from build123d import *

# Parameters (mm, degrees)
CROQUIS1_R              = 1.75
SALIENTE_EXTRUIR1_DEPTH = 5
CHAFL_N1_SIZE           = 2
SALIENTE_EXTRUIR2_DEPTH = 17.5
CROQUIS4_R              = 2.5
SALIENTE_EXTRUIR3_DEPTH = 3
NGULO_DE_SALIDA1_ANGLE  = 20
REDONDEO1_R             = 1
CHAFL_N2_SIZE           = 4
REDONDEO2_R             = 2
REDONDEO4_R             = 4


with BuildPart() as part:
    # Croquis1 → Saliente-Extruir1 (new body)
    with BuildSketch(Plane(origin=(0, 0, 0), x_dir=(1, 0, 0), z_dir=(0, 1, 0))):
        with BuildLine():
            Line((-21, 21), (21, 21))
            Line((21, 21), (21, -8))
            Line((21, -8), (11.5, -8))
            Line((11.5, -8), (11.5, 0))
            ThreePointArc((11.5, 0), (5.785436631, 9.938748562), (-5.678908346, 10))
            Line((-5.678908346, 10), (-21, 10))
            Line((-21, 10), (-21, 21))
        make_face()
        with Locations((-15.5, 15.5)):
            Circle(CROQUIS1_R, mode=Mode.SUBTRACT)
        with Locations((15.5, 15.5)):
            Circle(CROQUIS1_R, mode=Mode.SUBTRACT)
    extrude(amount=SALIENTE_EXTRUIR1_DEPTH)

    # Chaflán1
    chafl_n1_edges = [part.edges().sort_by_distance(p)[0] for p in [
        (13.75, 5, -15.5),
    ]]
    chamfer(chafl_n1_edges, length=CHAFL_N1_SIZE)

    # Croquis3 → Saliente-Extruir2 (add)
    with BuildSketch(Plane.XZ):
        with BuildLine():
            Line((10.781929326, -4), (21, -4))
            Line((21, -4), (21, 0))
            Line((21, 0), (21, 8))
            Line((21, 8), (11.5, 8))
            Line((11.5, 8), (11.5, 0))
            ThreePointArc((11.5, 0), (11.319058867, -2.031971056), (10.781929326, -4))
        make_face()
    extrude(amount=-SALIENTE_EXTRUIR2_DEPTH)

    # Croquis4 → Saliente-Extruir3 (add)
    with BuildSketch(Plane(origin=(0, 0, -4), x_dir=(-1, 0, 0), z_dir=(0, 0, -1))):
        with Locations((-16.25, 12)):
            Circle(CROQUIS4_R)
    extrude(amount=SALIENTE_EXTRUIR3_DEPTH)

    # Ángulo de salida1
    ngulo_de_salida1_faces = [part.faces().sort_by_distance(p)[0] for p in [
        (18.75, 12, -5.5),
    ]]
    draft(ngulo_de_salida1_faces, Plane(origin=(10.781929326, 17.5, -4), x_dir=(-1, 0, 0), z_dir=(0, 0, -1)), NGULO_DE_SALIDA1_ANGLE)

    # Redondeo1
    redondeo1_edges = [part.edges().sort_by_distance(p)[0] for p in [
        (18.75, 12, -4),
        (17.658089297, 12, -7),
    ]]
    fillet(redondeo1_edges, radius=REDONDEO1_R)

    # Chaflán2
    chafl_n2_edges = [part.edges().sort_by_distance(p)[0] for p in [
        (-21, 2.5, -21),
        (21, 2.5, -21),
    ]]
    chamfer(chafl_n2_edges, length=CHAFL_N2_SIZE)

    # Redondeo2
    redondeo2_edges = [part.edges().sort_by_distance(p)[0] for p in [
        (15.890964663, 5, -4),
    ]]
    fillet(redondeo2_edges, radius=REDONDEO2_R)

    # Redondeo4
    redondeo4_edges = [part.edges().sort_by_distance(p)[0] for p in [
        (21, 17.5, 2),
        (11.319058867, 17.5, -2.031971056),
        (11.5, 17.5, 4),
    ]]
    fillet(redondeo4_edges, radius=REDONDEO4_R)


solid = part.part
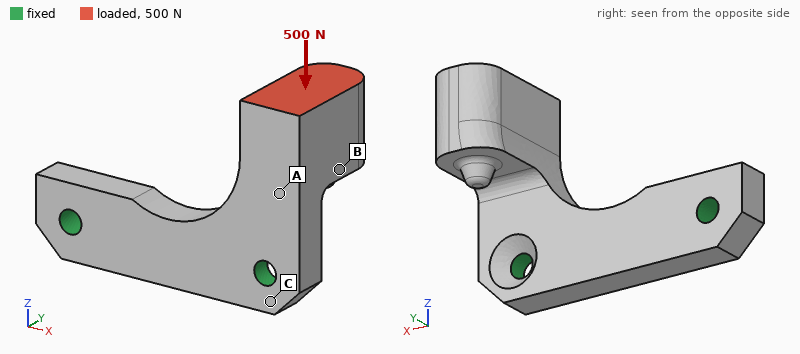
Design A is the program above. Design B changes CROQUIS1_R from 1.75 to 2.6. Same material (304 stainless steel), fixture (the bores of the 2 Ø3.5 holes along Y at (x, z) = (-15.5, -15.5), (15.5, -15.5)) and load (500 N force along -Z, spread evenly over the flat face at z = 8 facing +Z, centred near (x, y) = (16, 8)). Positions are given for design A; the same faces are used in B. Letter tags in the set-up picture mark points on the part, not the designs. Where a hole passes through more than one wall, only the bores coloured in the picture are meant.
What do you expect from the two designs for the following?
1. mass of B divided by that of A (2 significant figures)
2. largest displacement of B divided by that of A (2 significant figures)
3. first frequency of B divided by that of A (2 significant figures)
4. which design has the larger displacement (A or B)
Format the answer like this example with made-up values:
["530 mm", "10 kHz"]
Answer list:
["0.97", "0.90", "1.1", "A"]
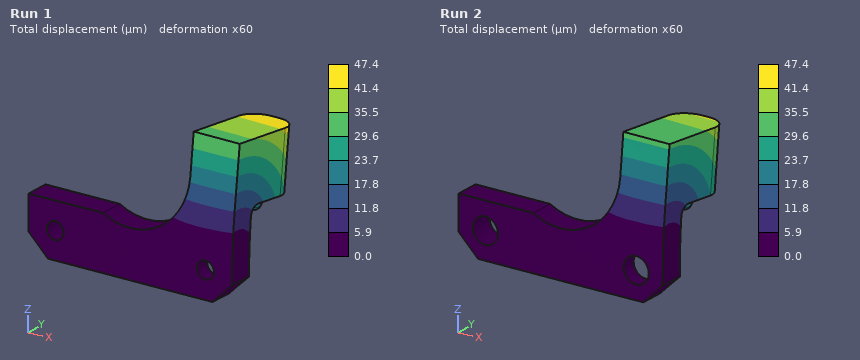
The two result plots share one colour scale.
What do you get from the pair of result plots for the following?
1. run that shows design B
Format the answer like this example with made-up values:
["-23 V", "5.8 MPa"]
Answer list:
["Run 2"]
